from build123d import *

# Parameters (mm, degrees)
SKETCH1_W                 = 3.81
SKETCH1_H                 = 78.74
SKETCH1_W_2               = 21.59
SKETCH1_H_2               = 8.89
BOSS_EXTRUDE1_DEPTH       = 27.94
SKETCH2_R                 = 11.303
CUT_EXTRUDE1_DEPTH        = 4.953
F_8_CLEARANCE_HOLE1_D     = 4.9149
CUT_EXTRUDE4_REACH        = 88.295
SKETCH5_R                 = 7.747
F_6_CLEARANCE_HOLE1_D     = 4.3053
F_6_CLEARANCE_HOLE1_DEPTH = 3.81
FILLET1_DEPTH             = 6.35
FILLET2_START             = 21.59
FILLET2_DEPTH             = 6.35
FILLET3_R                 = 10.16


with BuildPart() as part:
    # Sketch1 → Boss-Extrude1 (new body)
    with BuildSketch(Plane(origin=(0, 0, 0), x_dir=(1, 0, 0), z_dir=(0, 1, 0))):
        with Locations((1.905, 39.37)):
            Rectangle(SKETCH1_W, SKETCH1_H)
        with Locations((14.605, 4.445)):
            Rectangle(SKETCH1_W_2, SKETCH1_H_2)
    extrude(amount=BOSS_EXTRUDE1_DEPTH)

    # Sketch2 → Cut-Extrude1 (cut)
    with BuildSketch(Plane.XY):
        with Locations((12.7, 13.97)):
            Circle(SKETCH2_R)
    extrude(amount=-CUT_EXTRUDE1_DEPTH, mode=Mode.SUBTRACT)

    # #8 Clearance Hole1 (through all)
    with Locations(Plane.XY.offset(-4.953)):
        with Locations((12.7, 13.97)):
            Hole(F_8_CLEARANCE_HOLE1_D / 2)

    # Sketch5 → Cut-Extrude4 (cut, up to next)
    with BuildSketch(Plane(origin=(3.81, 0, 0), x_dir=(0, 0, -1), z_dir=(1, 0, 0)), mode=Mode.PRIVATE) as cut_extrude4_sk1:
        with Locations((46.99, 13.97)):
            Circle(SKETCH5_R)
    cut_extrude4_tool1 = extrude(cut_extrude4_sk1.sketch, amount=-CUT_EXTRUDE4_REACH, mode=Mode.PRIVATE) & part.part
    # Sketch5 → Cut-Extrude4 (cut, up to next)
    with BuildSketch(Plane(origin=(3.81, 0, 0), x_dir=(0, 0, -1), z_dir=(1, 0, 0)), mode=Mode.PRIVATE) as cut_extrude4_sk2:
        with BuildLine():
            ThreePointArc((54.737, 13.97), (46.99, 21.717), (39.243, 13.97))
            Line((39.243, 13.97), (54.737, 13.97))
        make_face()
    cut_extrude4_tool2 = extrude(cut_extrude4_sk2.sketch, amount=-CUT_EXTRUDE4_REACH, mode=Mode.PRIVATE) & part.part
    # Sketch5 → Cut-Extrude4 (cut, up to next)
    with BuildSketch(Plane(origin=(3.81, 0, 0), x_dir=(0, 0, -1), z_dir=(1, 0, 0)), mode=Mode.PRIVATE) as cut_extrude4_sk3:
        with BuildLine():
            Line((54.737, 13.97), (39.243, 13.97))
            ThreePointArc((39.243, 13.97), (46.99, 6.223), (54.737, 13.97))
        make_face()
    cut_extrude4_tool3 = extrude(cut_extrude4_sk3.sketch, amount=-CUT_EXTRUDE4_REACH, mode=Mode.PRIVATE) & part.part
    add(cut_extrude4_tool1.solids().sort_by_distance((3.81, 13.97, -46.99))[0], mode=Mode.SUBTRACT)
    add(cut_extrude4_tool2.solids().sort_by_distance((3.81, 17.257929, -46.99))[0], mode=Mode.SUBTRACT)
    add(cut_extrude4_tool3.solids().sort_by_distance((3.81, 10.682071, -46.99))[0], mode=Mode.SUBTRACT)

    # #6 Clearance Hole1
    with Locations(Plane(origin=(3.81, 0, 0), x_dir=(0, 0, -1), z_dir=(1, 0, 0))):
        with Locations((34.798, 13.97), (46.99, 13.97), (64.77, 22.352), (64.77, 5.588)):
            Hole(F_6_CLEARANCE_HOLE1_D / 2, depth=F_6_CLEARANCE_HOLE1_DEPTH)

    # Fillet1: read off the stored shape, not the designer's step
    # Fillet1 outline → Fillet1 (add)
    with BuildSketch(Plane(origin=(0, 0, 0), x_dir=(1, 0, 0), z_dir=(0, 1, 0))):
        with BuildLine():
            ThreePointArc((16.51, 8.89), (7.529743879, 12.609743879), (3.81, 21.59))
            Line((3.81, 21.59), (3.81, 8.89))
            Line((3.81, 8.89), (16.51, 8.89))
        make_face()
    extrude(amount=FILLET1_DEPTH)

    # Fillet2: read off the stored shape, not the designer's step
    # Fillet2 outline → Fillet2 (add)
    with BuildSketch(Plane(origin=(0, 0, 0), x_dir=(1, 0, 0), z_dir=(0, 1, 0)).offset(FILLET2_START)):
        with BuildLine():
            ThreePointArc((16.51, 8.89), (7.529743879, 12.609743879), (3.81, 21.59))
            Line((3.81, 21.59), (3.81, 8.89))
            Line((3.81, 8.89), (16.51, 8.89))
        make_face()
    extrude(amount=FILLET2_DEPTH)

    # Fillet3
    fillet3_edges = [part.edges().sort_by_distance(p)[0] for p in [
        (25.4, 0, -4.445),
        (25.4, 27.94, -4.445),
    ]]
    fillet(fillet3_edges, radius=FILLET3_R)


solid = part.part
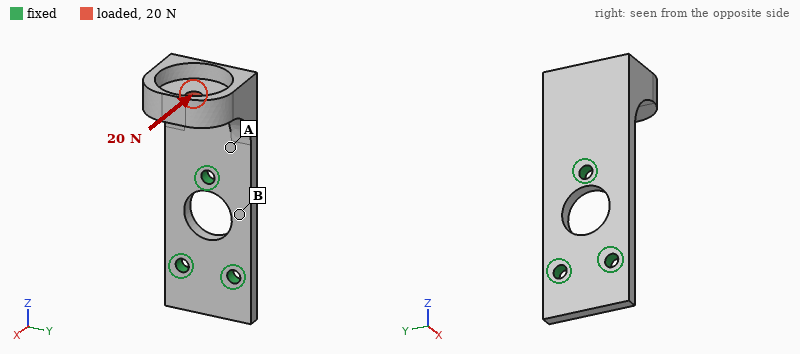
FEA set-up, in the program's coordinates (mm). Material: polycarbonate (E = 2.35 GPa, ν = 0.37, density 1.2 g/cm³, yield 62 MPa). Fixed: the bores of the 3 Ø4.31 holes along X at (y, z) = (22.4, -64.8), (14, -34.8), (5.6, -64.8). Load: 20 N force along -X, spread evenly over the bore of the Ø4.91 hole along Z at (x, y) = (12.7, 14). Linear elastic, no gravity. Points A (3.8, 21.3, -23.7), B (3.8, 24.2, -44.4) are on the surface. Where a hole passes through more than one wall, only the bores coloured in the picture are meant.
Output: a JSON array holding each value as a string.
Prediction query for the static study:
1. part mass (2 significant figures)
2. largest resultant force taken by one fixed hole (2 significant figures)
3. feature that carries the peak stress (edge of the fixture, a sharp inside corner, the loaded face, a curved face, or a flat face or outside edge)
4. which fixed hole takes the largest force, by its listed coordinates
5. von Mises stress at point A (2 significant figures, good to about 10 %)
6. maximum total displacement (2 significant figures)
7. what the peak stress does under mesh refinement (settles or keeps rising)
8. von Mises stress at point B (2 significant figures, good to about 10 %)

["13 g", "26 N", "edge of the fixture", "(14, -34.8)", "4.6 MPa", "0.84 mm", "keeps rising", "1.4 MPa"]
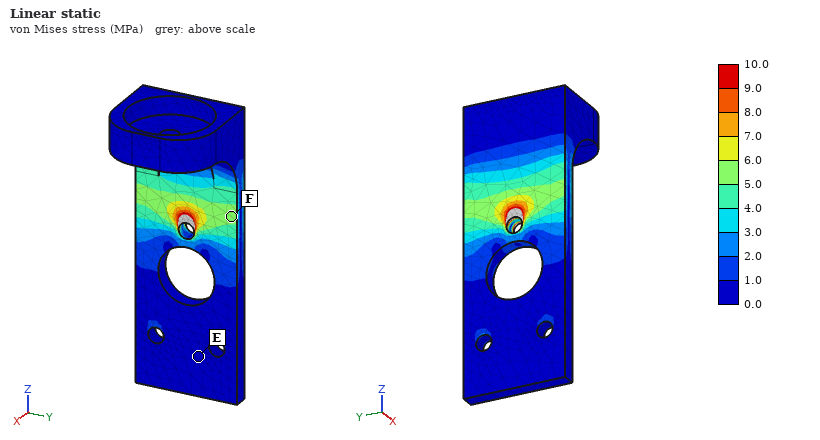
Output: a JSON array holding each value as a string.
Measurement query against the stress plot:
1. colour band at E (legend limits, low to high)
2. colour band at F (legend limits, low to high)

["0.0 to 1.0 MPa", "5.0 to 6.0 MPa"]
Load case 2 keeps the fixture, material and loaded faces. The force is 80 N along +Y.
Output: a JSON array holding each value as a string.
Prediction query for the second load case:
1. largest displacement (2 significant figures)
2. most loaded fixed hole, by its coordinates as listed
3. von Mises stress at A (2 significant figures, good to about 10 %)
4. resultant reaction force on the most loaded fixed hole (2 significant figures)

["1.0 mm", "(14, -34.8)", "9.1 MPa", "110 N"]
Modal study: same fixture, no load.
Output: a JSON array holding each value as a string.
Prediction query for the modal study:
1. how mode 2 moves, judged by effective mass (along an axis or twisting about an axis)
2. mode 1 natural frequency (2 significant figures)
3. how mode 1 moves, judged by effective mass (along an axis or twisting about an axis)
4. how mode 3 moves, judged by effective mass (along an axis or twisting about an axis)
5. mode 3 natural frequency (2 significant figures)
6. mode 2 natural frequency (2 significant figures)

["along Y", "360 Hz", "along X", "along Y", "1700 Hz", "670 Hz"]
